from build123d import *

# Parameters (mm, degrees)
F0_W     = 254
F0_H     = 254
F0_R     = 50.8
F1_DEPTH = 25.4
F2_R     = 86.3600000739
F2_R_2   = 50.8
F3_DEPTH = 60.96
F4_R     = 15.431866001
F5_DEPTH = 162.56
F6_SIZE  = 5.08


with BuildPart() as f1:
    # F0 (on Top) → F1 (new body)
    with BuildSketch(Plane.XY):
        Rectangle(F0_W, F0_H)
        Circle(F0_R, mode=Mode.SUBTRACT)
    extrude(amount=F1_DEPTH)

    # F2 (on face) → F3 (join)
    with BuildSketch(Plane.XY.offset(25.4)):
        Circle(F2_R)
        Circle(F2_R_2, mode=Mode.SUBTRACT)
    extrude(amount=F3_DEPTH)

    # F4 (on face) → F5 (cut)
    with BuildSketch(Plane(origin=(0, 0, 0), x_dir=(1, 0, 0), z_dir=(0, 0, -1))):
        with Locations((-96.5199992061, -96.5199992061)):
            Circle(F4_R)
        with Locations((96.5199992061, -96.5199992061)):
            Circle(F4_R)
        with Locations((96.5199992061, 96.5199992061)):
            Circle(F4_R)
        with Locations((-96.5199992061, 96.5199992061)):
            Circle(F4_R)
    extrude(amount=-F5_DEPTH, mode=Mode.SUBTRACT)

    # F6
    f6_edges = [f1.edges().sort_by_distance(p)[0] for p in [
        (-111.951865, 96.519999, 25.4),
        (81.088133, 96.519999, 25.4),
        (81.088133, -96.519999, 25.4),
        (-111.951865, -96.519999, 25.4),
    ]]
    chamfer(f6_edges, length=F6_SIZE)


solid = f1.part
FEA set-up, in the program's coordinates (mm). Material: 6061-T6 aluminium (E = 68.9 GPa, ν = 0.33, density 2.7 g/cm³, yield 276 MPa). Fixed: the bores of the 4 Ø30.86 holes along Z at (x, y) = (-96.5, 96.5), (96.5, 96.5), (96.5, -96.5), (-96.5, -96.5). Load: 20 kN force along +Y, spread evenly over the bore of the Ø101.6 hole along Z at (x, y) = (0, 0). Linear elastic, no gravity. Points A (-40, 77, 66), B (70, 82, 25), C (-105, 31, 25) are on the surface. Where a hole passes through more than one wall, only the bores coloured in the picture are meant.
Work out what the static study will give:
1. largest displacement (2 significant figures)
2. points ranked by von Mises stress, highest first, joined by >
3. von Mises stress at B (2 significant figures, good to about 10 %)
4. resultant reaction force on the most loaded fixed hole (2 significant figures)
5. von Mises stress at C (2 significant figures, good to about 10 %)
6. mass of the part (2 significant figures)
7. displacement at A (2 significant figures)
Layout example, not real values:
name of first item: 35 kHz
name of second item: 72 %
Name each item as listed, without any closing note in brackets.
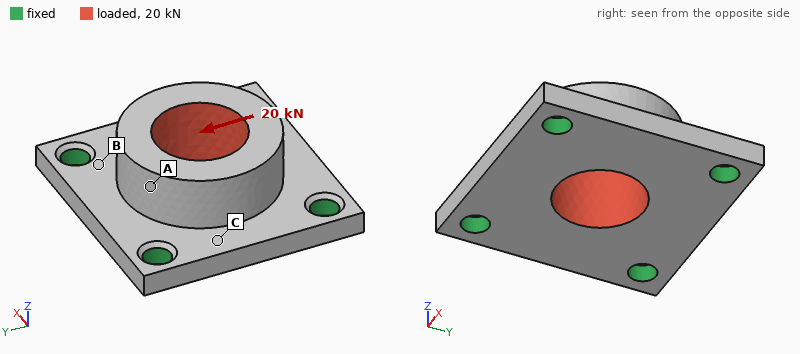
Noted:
largest displacement: 12 µm
points ranked by von Mises stress, highest first, joined by >: B > C > A
von Mises stress at B: 3.8 MPa
resultant reaction force on the most loaded fixed hole: 5.7 kN
von Mises stress at C: 2.4 MPa
mass of the part: 6.2 kg
displacement at A: 9.4 µm
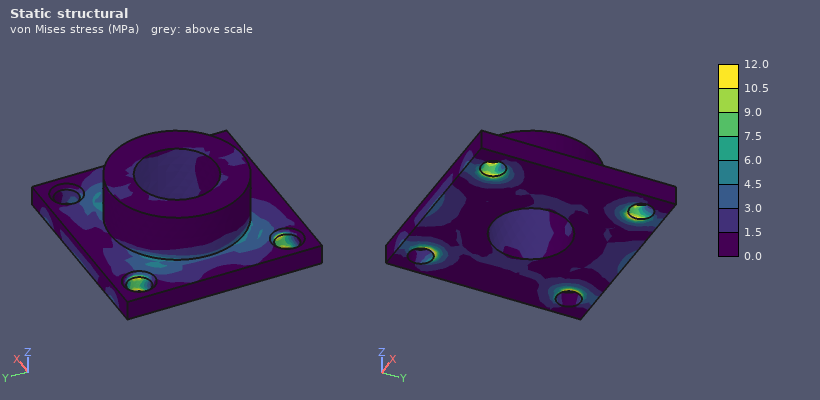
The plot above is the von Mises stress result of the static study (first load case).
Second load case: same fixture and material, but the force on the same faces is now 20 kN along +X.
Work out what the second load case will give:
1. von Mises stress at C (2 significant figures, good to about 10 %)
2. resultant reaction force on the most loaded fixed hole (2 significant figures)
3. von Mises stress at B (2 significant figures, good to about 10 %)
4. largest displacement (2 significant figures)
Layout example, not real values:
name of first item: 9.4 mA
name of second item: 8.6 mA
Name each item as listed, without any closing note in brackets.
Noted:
von Mises stress at C: 1.9 MPa
resultant reaction force on the most loaded fixed hole: 5.7 kN
von Mises stress at B: 4.2 MPa
largest displacement: 12 µm
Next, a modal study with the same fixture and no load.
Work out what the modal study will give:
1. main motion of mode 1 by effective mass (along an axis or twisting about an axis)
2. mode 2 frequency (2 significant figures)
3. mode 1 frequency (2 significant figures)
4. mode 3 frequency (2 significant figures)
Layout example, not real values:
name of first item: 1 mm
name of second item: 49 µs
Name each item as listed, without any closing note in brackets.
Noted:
main motion of mode 1 by effective mass: along Z
mode 2 frequency: 3200 Hz
mode 1 frequency: 2600 Hz
mode 3 frequency: 3200 Hz
